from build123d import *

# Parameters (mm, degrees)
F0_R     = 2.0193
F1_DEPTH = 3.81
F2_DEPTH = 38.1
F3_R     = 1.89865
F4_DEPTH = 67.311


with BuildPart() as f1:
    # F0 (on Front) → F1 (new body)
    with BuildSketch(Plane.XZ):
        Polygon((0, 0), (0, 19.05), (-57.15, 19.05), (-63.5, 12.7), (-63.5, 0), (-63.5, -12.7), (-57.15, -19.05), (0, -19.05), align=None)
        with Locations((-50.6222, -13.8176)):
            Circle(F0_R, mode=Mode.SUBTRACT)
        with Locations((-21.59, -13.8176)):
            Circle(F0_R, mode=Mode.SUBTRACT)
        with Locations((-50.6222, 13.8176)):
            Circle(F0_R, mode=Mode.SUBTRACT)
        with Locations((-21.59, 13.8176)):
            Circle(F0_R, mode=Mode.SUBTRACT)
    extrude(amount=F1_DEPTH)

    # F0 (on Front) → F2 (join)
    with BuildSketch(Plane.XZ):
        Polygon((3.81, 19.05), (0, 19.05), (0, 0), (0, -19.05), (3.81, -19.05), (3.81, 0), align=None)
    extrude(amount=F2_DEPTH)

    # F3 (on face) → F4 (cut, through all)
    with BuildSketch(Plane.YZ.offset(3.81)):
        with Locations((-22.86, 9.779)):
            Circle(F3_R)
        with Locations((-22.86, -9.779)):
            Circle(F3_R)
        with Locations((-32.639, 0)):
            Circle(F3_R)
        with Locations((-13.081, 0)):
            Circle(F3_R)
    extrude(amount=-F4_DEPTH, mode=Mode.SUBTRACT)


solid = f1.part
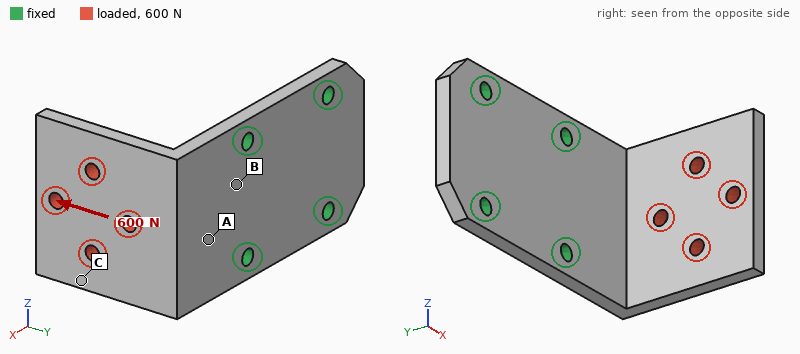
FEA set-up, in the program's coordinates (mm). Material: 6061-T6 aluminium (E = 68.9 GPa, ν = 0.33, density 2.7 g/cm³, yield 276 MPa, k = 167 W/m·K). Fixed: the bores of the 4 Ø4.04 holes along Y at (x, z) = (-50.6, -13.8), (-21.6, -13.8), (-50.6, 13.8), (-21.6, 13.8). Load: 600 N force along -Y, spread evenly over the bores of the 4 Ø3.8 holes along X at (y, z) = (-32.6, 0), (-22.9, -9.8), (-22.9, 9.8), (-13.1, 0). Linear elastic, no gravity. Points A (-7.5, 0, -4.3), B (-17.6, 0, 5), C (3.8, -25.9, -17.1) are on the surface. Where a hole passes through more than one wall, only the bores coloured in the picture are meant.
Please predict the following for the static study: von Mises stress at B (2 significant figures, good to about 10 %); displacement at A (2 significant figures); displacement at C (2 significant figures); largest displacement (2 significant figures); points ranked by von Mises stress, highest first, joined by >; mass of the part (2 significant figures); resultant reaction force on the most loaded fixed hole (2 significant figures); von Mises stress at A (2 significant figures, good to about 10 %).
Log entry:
84 MPa
0.10 mm
0.40 mm
0.54 mm
B > A > C
38 g
350 N
56 MPa
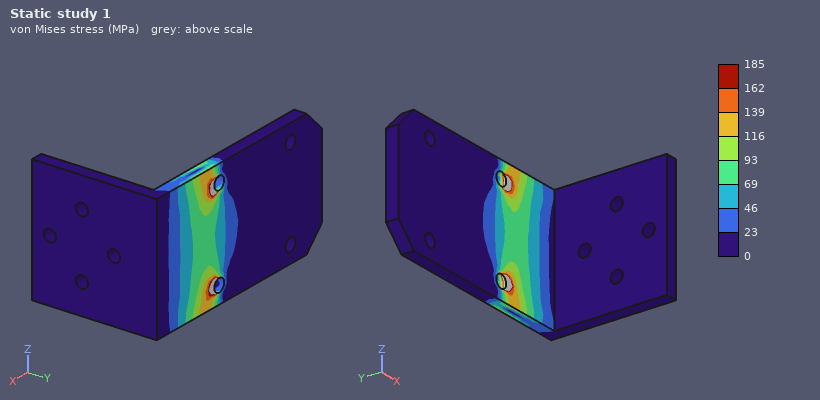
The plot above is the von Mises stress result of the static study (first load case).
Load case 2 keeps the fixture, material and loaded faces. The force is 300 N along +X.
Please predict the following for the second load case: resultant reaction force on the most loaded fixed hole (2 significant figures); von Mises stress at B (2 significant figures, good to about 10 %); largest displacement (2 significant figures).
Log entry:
140 N
47 MPa
0.59 mm
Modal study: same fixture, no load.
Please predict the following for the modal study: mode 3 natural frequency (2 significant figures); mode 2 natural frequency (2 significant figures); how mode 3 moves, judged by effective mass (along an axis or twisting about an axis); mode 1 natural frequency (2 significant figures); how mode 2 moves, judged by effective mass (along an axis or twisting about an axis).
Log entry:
3400 Hz
2300 Hz
along Y
1200 Hz
along Z
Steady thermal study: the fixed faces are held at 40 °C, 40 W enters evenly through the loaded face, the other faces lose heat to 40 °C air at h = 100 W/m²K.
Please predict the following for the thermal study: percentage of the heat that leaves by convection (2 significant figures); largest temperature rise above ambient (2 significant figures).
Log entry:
39 %
54 K
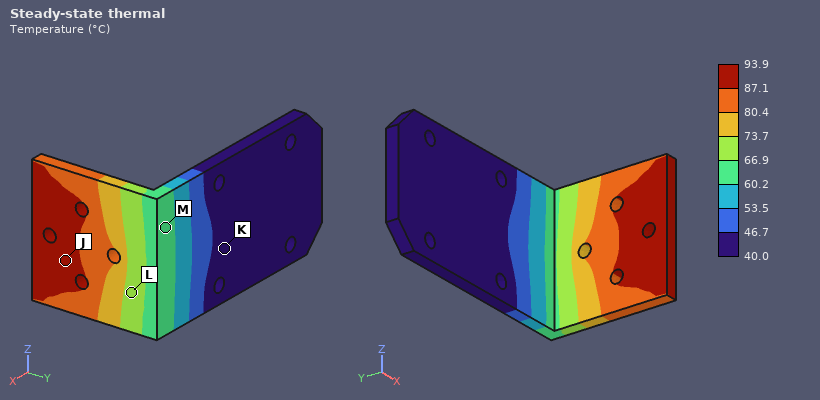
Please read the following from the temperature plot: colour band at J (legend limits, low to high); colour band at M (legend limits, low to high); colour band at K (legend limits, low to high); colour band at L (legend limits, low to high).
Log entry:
87.1 to 93.9 °C
60.2 to 66.9 °C
40.0 to 46.7 °C
66.9 to 73.7 °C
